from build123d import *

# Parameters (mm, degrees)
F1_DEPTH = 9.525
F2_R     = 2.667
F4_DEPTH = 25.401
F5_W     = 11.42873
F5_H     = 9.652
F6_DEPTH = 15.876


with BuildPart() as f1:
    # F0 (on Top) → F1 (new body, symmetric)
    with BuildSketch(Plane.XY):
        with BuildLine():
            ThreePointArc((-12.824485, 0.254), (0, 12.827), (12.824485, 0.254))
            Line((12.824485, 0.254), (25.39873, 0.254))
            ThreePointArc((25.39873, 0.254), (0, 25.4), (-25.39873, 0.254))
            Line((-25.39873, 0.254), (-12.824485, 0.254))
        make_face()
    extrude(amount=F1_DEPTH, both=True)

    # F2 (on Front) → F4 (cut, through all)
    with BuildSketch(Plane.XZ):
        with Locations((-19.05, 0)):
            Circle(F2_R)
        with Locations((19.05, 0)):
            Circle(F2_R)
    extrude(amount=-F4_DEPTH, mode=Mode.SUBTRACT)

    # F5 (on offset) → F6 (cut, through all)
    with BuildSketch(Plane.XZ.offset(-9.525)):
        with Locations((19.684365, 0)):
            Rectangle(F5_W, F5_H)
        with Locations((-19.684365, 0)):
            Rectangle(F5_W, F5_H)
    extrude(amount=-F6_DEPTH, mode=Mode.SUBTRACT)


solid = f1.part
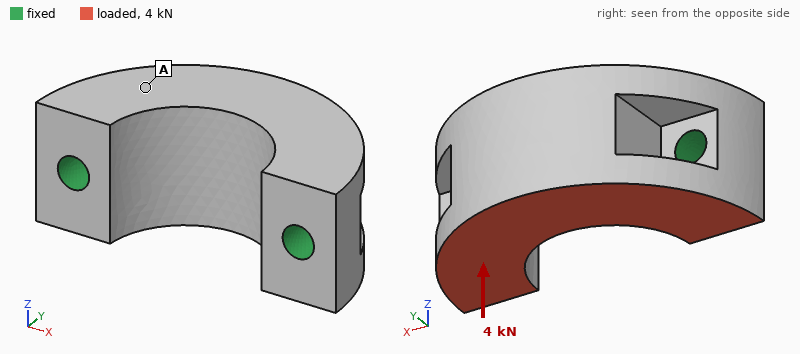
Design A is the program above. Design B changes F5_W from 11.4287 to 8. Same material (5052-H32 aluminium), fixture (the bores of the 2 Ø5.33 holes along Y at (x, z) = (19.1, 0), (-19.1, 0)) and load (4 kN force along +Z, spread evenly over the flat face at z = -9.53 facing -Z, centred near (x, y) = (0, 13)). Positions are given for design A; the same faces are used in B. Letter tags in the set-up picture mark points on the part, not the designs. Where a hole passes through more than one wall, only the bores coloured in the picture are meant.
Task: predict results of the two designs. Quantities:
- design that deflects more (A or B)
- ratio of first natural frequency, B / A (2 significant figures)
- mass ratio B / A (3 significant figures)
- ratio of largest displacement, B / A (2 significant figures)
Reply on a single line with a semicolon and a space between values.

A; 1.1; 1.03; 0.88
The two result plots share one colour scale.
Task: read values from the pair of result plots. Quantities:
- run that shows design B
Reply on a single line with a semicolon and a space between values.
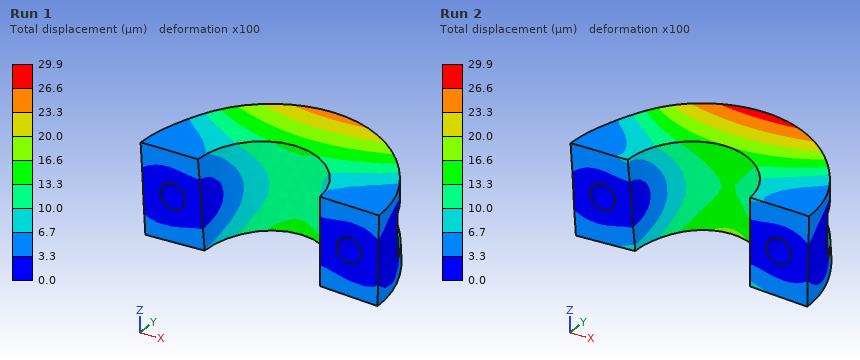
Run 1
